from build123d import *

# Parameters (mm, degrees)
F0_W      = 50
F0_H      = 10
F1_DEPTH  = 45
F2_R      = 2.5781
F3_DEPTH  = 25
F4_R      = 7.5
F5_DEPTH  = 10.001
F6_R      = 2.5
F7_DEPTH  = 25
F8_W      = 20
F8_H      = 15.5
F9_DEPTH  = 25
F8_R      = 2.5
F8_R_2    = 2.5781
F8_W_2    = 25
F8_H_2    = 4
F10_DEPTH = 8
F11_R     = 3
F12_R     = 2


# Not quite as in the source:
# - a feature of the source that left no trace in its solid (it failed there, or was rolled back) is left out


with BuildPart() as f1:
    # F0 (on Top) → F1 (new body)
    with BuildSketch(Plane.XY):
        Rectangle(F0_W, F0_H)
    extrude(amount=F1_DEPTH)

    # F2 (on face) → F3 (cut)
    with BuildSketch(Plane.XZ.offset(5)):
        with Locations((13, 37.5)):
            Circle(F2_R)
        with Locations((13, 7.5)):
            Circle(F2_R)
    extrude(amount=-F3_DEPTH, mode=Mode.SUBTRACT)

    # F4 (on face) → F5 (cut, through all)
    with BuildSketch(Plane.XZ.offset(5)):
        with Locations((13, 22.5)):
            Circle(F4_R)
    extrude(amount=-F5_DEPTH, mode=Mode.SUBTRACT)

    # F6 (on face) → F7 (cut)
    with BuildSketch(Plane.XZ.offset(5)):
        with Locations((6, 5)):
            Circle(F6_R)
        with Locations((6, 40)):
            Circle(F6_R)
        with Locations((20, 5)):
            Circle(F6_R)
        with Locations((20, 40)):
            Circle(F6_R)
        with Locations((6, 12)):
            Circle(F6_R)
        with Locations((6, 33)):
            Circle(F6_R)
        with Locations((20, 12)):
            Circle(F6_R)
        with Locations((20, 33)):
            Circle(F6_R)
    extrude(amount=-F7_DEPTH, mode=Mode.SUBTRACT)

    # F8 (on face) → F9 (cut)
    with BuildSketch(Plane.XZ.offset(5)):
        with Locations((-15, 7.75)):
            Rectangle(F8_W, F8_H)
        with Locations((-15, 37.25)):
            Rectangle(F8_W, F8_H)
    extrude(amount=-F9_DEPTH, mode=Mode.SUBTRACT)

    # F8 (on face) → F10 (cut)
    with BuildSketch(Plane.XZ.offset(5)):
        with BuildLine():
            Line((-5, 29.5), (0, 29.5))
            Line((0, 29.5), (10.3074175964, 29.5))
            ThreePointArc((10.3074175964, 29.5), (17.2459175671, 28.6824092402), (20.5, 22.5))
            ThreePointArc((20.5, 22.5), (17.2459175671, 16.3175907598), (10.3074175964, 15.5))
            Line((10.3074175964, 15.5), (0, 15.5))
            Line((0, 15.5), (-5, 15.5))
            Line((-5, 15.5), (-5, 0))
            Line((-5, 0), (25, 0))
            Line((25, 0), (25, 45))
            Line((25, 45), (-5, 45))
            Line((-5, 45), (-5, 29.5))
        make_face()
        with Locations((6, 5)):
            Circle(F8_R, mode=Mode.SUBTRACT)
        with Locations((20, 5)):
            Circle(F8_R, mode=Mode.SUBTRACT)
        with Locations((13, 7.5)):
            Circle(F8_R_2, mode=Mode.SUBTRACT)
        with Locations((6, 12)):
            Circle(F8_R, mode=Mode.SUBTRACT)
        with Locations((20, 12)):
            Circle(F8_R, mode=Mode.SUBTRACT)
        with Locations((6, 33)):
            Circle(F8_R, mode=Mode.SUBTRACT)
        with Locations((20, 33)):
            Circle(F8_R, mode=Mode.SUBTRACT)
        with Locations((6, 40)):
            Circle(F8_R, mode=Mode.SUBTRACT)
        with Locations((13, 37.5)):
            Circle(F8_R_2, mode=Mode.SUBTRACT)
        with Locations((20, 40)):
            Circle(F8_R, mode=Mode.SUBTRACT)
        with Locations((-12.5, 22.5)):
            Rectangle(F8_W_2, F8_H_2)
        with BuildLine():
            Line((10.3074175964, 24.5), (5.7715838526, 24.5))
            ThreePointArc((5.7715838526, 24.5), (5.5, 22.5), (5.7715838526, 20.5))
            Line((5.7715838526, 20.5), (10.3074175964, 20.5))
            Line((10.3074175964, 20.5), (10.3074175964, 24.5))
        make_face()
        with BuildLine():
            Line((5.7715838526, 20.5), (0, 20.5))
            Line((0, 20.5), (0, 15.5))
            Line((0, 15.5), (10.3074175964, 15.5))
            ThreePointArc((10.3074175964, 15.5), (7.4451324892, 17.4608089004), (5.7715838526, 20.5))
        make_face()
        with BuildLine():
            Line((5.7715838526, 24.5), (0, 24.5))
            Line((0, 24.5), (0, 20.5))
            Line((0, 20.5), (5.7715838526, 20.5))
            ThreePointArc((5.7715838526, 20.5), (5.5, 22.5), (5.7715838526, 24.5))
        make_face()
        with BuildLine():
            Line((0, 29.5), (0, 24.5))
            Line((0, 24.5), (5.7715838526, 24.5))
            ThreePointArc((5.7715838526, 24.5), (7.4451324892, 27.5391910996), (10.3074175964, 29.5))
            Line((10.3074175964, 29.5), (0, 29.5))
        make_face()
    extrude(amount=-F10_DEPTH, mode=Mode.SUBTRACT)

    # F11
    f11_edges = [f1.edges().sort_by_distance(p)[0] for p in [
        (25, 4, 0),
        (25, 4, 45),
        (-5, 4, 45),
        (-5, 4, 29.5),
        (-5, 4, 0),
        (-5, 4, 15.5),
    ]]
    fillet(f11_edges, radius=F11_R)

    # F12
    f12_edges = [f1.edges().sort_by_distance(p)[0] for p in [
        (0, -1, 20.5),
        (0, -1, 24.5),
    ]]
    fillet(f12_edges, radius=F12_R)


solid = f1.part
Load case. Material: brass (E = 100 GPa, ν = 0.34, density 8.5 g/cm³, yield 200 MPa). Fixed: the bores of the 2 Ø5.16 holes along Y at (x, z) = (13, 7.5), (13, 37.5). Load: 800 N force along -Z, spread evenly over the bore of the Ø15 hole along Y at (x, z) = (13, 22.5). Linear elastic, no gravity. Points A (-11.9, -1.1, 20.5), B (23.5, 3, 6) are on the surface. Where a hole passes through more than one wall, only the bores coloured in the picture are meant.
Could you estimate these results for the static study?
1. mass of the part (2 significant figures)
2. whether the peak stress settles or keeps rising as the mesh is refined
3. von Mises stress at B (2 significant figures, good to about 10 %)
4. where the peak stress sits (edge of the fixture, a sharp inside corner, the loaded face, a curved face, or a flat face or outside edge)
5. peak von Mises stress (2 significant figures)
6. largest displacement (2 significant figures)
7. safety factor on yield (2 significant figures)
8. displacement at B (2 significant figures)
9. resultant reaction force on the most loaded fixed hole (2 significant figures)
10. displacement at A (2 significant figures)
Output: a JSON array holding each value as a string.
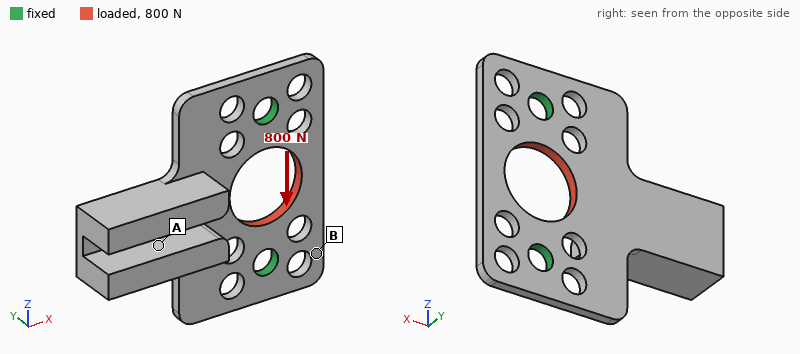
["38 g", "settles", "8.4 MPa", "a curved face", "58 MPa", "4.1 µm", "3.5", "2.4 µm", "400 N", "1.4 µm"]
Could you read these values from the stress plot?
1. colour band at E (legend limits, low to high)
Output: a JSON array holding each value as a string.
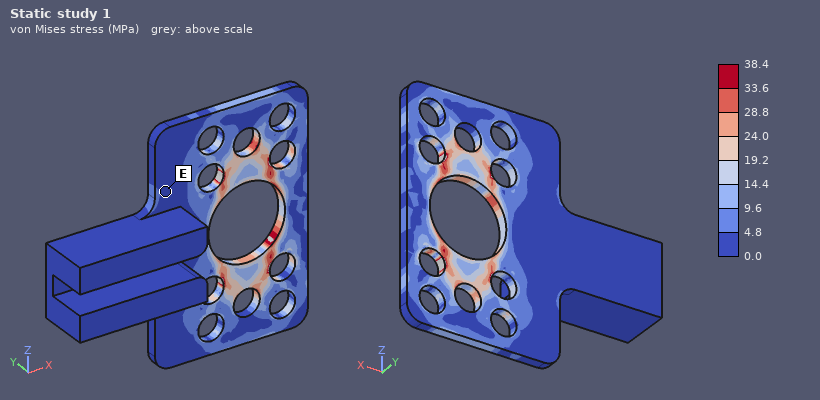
["0.0 to 4.8 MPa"]
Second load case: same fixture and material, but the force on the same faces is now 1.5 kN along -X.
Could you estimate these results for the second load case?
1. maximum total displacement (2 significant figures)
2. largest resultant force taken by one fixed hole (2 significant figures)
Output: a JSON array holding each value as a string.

["11 µm", "750 N"]
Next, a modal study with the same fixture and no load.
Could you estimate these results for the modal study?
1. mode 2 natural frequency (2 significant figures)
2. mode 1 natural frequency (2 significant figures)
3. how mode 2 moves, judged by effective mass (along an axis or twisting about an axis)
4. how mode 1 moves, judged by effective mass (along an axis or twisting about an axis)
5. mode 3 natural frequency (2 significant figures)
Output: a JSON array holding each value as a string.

["2900 Hz", "520 Hz", "along Z", "along Y", "4300 Hz"]
